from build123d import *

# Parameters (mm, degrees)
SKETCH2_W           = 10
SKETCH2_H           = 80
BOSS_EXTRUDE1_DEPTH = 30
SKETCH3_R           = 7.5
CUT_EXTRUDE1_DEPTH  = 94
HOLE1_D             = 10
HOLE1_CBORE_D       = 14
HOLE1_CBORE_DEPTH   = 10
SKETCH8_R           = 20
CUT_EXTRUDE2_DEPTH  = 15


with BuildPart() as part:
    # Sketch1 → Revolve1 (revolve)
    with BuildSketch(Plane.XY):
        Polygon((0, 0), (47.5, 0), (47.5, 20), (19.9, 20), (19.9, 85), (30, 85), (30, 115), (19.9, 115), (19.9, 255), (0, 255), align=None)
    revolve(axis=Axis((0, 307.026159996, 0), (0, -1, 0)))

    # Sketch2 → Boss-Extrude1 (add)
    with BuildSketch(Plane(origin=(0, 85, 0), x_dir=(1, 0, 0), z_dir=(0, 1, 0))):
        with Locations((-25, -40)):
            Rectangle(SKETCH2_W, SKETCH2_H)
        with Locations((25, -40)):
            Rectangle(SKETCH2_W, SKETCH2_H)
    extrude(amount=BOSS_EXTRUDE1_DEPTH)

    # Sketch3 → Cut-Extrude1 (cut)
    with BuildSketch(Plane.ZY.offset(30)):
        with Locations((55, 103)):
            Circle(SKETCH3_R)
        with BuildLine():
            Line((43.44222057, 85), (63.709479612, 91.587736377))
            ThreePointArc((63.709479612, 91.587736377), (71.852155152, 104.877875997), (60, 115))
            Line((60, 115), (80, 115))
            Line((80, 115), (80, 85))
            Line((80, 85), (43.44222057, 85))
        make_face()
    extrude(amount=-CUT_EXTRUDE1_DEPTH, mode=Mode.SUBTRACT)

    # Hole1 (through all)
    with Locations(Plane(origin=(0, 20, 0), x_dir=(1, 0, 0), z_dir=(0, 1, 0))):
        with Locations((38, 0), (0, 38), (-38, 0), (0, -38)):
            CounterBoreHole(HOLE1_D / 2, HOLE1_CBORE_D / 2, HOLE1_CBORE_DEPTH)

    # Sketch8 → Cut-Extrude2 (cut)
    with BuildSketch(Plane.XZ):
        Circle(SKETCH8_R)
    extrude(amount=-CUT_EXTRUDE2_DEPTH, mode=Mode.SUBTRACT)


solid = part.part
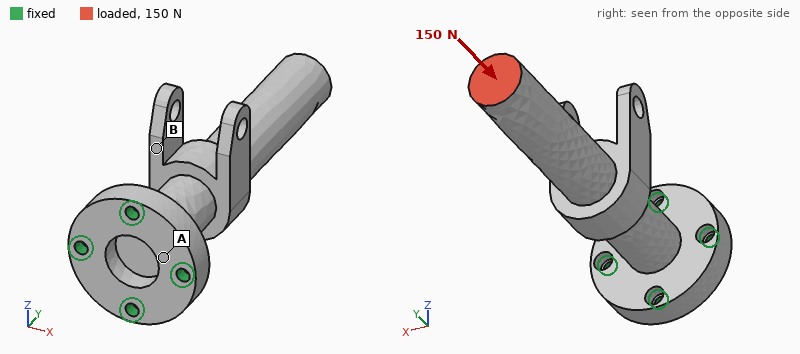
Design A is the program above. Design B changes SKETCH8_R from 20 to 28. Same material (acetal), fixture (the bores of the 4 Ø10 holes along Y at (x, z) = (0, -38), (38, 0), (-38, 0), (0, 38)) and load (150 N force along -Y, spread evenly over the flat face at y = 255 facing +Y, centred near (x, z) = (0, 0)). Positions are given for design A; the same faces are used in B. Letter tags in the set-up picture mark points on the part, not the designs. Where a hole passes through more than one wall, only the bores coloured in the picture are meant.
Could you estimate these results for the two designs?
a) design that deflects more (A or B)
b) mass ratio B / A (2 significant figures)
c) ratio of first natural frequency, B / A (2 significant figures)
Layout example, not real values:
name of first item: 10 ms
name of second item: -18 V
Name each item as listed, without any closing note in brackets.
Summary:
design that deflects more: B
mass ratio B / A: 0.96
ratio of first natural frequency, B / A: 0.83
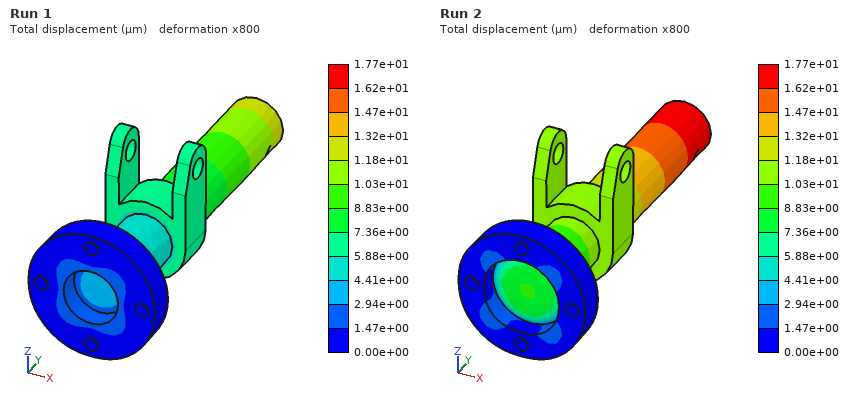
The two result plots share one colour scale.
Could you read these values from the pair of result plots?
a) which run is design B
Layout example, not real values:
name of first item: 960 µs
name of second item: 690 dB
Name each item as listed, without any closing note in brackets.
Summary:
which run is design B: Run 2
